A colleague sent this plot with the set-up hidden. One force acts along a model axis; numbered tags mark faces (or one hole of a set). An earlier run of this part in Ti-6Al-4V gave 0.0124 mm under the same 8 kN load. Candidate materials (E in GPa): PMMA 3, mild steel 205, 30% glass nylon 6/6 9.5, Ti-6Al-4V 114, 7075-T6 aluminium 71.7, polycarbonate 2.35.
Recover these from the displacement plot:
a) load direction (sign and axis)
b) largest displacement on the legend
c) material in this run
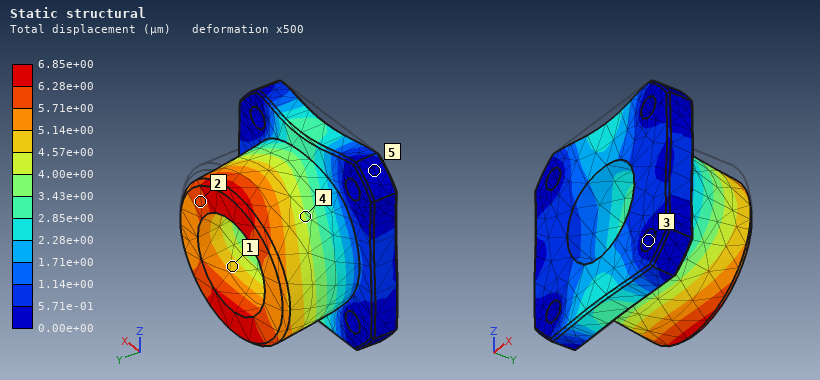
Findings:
-Z
6.85e+00 µm
mild steel
